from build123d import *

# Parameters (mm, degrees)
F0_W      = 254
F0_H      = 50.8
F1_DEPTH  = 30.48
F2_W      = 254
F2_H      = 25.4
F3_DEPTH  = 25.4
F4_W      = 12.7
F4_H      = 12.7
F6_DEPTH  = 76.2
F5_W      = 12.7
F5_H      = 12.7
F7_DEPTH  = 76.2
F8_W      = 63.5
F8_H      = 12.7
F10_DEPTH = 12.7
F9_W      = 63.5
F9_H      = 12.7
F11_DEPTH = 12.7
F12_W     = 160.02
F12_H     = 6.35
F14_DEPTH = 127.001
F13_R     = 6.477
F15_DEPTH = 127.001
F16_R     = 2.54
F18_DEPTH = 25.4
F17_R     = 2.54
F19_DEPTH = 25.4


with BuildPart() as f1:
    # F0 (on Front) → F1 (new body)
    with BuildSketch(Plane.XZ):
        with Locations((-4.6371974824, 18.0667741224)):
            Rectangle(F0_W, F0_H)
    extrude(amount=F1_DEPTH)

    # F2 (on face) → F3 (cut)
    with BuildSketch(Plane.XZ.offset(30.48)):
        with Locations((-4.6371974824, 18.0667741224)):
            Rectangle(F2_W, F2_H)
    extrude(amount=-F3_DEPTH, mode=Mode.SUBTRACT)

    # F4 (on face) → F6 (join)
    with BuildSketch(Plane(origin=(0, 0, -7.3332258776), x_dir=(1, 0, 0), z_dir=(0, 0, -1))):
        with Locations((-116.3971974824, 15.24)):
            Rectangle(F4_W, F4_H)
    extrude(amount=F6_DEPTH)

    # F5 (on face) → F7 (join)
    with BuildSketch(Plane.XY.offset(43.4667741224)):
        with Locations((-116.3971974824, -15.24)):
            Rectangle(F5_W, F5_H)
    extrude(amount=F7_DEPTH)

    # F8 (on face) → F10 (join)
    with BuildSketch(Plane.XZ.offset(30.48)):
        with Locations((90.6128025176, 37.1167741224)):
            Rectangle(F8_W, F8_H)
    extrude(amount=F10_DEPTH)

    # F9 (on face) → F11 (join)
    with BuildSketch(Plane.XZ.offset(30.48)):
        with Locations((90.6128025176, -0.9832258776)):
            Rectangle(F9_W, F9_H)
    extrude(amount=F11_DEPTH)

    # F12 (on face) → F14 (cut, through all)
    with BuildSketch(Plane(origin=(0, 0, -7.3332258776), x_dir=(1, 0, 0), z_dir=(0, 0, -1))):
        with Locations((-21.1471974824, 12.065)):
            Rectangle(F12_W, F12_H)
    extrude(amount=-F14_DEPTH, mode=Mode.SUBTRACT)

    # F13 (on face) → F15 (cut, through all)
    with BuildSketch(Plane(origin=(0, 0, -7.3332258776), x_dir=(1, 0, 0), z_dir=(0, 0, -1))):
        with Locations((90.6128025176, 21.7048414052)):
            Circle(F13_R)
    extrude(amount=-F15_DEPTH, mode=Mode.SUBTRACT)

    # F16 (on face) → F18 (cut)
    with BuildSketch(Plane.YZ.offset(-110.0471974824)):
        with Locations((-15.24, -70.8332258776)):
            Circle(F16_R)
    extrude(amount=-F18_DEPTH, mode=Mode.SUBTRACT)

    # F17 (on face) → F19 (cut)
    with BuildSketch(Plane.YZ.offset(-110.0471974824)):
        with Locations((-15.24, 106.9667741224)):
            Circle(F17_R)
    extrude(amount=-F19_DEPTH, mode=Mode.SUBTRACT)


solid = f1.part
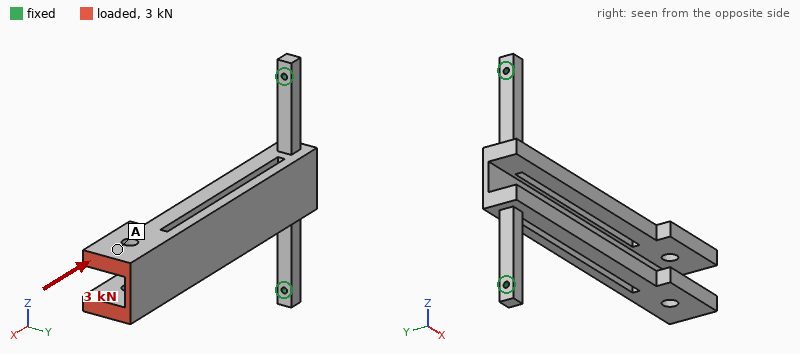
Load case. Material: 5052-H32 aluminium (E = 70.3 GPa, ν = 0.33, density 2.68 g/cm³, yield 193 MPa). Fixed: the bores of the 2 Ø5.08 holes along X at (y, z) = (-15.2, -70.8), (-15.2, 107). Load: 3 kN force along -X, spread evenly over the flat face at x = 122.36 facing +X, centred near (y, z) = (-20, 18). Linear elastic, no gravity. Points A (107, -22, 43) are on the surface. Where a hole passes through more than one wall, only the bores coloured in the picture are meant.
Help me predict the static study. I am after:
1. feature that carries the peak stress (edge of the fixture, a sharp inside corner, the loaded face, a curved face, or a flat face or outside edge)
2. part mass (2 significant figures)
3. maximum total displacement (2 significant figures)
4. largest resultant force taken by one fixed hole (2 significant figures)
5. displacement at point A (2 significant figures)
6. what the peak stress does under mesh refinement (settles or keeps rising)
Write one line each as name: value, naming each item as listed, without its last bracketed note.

feature that carries the peak stress: edge of the fixture
part mass: 660 g
maximum total displacement: 1.2 mm
largest resultant force taken by one fixed hole: 1.5 kN
displacement at point A: 1.1 mm
what the peak stress does under mesh refinement: keeps rising
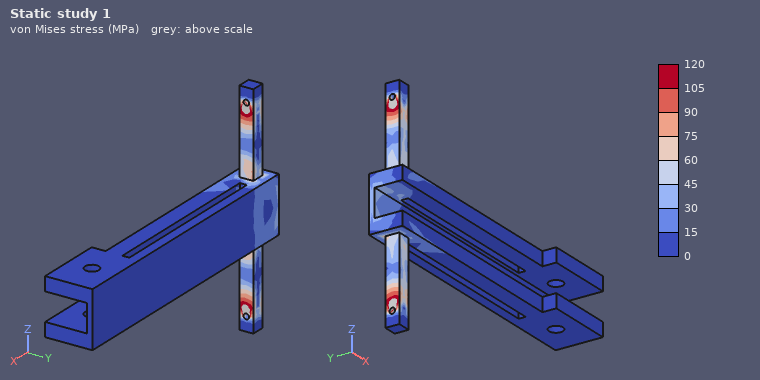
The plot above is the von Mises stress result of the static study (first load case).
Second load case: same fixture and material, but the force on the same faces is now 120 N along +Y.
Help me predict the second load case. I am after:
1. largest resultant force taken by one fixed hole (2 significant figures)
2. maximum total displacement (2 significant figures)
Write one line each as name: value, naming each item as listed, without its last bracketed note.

largest resultant force taken by one fixed hole: 150 N
maximum total displacement: 2.4 mm
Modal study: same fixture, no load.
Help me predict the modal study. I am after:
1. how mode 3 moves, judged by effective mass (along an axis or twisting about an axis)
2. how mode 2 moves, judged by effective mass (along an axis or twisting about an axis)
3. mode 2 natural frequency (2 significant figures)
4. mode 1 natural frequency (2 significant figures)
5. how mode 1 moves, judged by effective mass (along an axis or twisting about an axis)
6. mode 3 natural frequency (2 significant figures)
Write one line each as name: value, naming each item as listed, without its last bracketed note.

how mode 3 moves, judged by effective mass: twisting about X
how mode 2 moves, judged by effective mass: along Z
mode 2 natural frequency: 240 Hz
mode 1 natural frequency: 77 Hz
how mode 1 moves, judged by effective mass: along Y
mode 3 natural frequency: 640 Hz
